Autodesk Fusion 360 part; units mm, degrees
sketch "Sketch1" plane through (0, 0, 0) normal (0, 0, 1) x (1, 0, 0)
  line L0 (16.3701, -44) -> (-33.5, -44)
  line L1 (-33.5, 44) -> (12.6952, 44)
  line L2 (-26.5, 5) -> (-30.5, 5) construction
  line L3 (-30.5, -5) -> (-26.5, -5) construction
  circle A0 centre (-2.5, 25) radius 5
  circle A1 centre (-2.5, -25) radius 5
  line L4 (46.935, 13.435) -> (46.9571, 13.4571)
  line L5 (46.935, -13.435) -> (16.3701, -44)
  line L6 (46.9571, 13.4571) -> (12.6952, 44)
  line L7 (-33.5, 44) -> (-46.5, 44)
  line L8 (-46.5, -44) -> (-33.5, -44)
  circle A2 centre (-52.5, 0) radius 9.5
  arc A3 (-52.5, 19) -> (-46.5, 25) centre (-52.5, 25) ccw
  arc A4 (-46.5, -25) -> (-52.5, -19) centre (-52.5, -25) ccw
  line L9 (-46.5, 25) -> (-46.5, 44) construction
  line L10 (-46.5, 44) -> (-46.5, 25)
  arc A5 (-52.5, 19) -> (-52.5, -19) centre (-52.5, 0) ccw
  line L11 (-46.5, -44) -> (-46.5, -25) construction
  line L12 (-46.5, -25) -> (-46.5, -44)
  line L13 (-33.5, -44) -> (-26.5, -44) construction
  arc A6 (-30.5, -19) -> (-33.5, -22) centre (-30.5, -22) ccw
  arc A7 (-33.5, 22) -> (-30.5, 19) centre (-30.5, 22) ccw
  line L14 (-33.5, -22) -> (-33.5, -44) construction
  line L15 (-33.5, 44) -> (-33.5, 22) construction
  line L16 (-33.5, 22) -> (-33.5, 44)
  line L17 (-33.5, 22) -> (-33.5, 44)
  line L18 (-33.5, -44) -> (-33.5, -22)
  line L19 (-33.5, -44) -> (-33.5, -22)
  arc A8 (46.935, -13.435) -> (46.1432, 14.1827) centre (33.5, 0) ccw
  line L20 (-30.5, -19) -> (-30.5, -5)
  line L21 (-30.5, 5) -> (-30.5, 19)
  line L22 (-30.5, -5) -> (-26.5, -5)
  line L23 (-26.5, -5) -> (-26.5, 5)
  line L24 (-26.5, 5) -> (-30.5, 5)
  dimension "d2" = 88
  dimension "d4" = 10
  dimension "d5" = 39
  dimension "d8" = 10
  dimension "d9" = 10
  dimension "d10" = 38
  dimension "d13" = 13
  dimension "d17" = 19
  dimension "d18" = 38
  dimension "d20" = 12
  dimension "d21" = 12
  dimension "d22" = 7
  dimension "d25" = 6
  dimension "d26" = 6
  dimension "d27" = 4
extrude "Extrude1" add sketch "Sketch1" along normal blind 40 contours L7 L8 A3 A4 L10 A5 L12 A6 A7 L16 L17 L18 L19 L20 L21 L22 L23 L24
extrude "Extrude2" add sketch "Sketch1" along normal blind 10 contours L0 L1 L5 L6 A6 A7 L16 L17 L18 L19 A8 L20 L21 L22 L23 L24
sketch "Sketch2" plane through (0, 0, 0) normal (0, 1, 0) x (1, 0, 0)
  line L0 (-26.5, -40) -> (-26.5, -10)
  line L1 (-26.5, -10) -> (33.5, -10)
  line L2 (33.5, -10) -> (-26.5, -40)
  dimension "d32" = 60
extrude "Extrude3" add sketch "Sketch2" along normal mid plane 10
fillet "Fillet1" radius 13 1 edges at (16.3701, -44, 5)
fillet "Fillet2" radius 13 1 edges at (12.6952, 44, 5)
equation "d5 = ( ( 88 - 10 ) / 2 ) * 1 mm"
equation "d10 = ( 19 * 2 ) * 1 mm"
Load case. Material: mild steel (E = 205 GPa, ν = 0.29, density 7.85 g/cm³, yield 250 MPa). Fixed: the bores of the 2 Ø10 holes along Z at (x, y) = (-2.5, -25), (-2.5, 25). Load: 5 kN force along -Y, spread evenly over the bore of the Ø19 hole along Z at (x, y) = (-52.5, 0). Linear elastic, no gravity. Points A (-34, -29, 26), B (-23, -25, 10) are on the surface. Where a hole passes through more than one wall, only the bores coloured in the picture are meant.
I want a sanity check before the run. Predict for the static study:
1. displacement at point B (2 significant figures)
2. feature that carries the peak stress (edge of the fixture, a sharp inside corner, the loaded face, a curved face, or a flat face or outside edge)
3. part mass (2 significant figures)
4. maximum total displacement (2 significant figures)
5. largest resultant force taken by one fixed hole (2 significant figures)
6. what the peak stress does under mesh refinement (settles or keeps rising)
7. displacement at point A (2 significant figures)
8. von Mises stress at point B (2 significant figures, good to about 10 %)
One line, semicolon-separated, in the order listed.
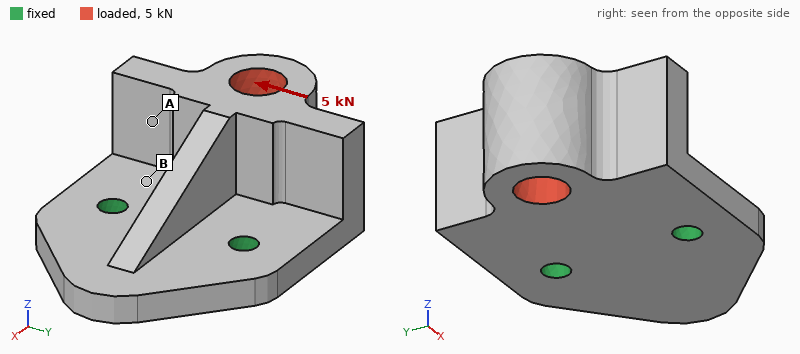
4.4 µm; edge of the fixture; 1.1 kg; 17 µm; 5.3 kN; keeps rising; 11 µm; 24 MPa
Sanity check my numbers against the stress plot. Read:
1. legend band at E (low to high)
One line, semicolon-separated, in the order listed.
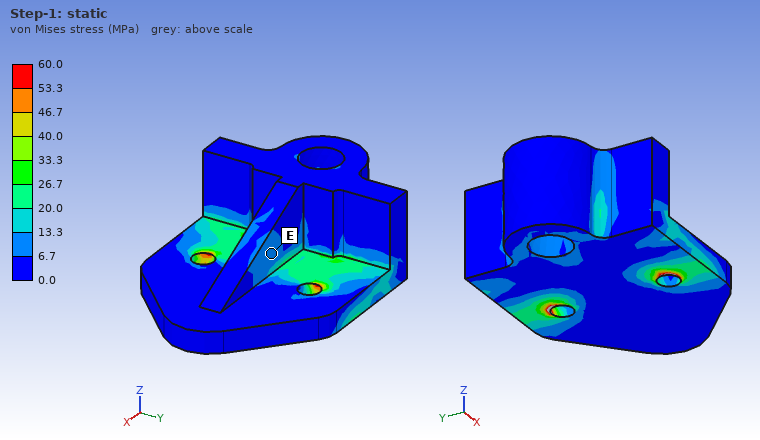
6.7 to 13.3 MPa
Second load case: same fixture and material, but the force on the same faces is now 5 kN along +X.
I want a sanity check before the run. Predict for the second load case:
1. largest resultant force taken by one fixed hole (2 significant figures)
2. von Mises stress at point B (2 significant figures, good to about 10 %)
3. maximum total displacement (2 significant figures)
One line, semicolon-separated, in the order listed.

2.5 kN; 16 MPa; 37 µm
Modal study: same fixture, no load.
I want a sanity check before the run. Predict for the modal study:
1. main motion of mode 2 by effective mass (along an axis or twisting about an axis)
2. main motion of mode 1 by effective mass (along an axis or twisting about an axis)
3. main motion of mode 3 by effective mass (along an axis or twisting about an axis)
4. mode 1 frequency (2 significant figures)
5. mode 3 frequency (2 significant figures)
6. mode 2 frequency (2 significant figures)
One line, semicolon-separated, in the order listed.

along Y; along Z; along Z; 1800 Hz; 5200 Hz; 3600 Hz
